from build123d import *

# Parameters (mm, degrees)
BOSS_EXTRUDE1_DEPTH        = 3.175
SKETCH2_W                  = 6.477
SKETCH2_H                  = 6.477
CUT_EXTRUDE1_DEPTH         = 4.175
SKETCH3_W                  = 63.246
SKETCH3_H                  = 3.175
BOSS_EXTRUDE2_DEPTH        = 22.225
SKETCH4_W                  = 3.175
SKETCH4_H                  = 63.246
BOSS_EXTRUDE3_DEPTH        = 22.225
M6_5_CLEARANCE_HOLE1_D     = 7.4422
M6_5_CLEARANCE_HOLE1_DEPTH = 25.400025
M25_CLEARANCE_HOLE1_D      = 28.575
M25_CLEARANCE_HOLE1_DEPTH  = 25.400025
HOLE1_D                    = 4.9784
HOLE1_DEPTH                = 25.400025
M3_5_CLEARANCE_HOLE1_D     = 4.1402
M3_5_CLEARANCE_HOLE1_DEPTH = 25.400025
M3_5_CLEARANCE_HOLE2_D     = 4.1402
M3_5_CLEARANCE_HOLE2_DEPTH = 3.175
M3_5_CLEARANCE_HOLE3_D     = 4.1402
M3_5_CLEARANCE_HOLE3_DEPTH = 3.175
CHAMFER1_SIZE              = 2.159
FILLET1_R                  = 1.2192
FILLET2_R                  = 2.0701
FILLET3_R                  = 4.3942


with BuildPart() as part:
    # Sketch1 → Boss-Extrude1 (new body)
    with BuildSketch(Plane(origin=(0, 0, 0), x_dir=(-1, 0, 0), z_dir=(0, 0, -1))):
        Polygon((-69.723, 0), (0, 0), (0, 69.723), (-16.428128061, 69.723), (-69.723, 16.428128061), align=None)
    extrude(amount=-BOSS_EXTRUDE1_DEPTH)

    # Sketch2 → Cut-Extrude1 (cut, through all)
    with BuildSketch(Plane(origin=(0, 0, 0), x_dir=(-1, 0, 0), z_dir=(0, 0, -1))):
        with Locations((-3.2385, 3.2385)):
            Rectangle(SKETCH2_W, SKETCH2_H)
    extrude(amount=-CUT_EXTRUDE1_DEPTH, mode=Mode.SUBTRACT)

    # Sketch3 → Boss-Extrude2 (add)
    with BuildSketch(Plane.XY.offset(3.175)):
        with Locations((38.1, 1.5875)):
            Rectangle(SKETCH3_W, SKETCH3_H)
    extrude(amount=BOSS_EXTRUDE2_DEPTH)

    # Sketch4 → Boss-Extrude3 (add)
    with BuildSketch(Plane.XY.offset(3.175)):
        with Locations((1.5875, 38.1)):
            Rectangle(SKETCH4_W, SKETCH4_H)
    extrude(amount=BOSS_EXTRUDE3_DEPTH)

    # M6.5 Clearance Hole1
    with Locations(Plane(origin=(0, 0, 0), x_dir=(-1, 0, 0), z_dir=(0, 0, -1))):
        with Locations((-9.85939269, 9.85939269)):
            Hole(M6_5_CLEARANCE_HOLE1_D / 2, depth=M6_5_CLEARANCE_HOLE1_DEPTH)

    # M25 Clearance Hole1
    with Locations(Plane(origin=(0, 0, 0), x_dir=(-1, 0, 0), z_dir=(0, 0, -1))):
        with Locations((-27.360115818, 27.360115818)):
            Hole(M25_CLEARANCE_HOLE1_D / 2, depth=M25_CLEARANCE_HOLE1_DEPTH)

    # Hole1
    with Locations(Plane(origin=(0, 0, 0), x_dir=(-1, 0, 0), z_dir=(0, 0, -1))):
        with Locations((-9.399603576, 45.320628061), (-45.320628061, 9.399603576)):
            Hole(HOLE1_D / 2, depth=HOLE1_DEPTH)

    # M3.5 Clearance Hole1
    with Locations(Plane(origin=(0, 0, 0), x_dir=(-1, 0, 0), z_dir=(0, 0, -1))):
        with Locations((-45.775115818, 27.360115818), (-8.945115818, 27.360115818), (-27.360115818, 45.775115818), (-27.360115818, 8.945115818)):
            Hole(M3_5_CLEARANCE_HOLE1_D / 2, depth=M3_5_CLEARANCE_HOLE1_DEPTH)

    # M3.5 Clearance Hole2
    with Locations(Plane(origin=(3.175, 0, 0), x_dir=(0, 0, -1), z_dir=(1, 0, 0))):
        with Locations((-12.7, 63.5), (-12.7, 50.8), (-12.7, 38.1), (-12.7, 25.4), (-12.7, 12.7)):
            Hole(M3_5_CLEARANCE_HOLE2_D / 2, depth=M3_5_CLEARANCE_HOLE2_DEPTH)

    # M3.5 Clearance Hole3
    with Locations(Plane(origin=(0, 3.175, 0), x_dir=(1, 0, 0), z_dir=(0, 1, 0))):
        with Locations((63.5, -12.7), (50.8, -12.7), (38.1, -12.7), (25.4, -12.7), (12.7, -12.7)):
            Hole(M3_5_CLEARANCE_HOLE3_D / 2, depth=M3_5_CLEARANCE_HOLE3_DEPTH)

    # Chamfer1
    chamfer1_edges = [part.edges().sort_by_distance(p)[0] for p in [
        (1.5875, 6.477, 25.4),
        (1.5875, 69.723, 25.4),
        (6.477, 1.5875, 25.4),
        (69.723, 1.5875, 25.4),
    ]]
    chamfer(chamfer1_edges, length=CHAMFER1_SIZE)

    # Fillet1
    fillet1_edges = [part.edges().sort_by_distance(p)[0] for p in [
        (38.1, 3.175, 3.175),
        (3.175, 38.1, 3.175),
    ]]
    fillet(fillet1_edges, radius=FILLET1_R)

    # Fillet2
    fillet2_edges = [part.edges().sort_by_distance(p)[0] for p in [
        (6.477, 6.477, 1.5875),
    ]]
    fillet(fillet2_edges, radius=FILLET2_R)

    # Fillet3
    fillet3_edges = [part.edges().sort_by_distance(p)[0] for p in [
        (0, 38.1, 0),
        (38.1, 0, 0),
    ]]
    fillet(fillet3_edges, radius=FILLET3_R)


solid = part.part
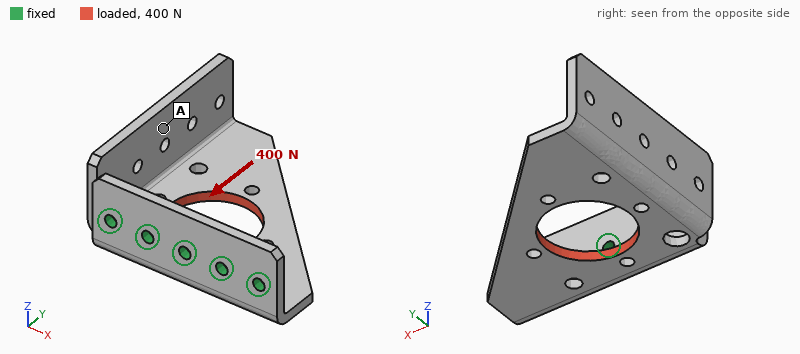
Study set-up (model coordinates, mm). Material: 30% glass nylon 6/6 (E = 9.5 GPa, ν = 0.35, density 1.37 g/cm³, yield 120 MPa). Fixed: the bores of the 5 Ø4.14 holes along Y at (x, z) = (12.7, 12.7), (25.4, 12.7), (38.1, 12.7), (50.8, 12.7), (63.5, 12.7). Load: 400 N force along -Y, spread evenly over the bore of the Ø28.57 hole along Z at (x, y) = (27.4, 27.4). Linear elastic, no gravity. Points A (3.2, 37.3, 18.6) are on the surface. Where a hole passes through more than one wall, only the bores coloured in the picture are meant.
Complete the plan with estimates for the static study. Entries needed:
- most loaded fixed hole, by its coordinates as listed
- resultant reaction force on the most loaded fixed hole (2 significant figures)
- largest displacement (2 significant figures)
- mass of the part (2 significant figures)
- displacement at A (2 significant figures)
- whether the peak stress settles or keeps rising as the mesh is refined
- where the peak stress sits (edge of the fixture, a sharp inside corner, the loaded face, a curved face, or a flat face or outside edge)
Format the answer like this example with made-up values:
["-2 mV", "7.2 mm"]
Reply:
["(12.7, 12.7)", "150 N", "1.1 mm", "22 g", "0.59 mm", "keeps rising", "edge of the fixture"]
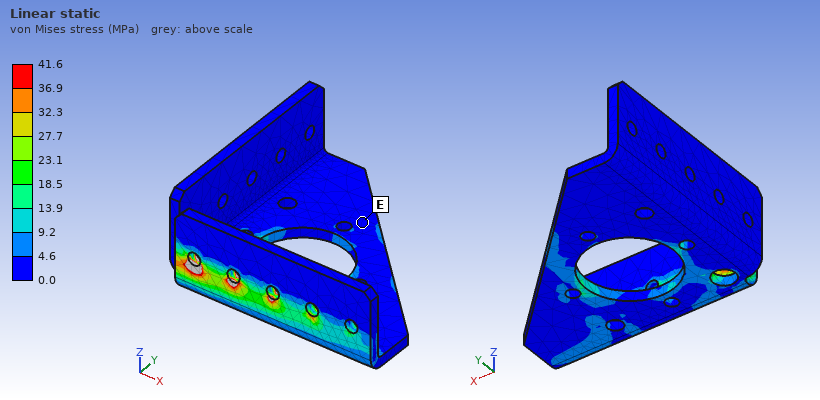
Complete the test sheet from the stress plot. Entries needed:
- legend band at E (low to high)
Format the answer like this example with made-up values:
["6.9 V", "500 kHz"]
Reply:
["0.0 to 4.6 MPa"]
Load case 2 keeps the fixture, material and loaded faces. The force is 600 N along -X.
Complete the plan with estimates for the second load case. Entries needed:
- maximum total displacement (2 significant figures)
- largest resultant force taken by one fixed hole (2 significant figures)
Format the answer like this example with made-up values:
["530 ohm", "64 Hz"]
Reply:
["1.2 mm", "290 N"]
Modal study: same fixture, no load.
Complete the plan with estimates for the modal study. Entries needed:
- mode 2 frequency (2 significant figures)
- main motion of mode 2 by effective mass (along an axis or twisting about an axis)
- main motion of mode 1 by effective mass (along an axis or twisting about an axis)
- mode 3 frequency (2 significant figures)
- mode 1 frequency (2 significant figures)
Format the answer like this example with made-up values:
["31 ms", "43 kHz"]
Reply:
["650 Hz", "along X", "along Z", "1200 Hz", "200 Hz"]
